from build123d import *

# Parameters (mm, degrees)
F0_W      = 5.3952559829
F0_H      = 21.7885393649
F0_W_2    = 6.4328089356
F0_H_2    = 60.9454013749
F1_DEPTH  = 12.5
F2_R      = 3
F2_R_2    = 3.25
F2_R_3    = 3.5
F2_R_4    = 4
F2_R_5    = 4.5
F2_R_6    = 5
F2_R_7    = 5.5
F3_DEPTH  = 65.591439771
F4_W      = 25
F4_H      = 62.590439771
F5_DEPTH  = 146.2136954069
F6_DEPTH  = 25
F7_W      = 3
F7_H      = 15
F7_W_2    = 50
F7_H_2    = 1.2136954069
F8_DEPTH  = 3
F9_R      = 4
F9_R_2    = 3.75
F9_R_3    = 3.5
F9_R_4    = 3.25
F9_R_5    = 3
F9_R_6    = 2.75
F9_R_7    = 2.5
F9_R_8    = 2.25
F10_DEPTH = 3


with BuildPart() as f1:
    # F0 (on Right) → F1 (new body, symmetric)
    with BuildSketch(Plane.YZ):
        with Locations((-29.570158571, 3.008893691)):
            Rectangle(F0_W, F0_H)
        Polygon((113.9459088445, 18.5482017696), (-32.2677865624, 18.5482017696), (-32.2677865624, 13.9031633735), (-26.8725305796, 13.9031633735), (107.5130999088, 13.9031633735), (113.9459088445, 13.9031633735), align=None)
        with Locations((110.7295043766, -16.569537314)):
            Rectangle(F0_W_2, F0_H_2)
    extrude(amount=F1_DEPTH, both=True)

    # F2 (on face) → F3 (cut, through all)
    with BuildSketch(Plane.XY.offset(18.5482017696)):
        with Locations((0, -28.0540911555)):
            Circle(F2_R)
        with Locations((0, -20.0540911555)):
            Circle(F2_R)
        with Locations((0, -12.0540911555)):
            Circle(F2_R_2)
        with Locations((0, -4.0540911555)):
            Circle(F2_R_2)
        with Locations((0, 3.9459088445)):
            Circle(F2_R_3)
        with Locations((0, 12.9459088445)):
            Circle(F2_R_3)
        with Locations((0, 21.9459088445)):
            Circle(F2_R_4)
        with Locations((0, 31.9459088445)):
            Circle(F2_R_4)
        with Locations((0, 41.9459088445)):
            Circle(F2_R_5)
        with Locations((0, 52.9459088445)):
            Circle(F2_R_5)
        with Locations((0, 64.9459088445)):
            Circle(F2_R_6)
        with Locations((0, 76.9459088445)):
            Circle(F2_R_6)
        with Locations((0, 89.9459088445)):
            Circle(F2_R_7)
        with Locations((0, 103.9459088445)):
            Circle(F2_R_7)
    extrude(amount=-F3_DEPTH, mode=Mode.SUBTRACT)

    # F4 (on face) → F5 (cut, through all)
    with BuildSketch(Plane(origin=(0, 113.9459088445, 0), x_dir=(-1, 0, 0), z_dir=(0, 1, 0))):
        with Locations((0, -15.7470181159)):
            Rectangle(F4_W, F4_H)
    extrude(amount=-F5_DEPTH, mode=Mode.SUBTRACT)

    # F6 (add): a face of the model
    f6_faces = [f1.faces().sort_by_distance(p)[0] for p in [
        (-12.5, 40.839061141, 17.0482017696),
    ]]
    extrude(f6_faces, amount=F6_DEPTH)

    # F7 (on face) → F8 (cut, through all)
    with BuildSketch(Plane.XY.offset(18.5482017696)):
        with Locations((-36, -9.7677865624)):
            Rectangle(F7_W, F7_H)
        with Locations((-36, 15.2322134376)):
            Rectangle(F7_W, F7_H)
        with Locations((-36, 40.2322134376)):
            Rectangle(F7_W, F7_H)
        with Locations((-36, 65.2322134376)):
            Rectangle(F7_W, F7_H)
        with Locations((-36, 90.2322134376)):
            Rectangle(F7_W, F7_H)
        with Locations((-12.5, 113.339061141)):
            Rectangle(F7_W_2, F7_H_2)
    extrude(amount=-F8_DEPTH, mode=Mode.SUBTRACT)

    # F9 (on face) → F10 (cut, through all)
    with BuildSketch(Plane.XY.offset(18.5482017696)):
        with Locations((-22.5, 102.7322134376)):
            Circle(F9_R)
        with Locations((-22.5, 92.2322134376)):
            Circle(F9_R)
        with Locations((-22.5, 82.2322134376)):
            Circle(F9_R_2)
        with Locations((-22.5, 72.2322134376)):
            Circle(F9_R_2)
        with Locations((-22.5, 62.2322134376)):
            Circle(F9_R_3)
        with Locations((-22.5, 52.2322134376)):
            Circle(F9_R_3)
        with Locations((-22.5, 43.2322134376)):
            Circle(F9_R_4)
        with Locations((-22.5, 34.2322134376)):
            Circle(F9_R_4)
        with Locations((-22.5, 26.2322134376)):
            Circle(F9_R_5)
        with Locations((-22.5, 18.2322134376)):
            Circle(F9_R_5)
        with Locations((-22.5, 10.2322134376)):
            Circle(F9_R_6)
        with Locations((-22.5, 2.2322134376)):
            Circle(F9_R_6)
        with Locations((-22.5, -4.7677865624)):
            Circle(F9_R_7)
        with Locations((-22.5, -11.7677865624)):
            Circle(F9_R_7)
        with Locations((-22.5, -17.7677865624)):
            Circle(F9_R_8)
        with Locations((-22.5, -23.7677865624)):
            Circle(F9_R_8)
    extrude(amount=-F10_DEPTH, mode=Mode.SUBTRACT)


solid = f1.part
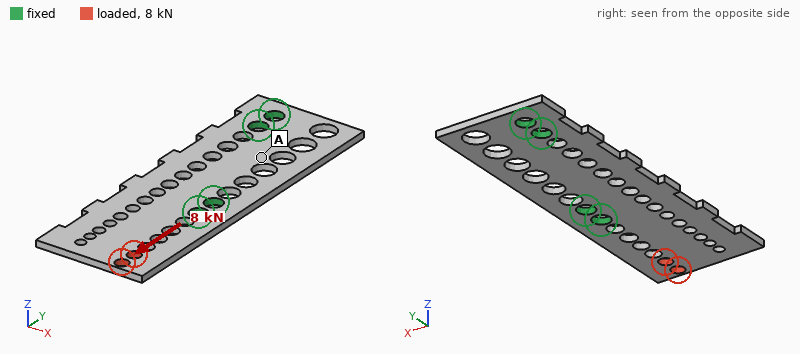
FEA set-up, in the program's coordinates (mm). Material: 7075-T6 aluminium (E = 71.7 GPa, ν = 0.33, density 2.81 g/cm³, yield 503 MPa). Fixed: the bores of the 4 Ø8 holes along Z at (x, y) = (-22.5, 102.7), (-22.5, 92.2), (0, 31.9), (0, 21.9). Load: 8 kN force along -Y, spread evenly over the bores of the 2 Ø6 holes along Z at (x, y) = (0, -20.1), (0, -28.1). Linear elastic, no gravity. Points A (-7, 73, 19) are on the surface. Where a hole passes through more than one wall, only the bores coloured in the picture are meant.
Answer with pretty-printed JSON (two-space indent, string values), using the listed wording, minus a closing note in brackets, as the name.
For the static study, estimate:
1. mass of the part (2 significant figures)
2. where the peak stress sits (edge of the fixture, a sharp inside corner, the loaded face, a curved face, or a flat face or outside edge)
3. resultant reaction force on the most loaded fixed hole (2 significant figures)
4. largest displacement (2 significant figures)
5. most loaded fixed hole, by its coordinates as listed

{
  "mass of the part": "48 g",
  "where the peak stress sits": "a flat face or outside edge",
  "resultant reaction force on the most loaded fixed hole": "5.6 kN",
  "largest displacement": "0.14 mm",
  "most loaded fixed hole, by its coordinates as listed": "(0, 21.9)"
}
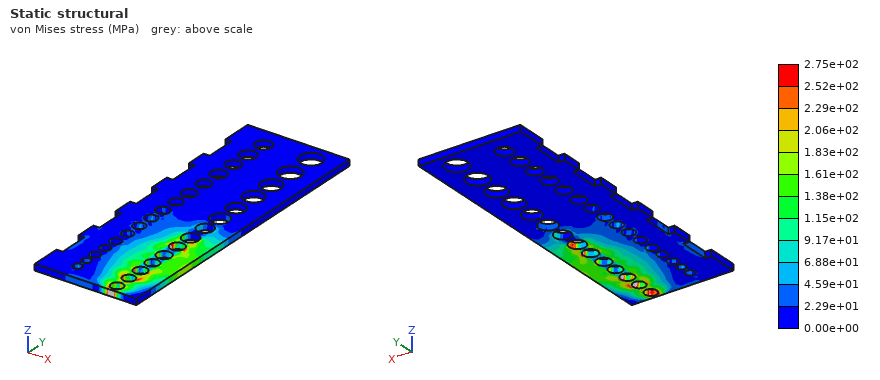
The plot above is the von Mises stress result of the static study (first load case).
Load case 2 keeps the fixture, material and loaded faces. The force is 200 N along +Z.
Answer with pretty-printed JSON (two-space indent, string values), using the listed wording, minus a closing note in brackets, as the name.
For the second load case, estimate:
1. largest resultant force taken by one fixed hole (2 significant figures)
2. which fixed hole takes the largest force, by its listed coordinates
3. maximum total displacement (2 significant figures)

{
  "largest resultant force taken by one fixed hole": "460 N",
  "which fixed hole takes the largest force, by its listed coordinates": "(0, 21.9)",
  "maximum total displacement": "1.5 mm"
}
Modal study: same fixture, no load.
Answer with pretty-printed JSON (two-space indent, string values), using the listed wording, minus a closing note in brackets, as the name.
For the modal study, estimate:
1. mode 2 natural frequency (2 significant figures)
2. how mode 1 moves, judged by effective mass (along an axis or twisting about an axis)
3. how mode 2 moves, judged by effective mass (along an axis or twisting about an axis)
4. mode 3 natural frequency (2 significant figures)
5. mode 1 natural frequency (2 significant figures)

{
  "mode 2 natural frequency": "1500 Hz",
  "how mode 1 moves, judged by effective mass": "along Z",
  "how mode 2 moves, judged by effective mass": "twisting about Y",
  "mode 3 natural frequency": "2400 Hz",
  "mode 1 natural frequency": "710 Hz"
}
